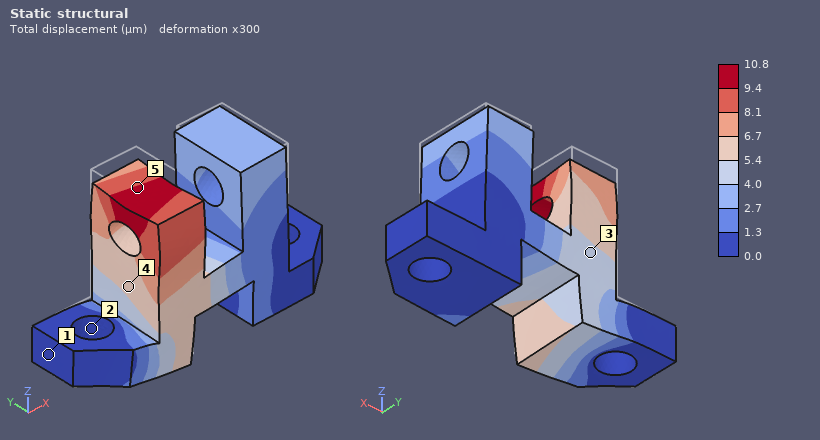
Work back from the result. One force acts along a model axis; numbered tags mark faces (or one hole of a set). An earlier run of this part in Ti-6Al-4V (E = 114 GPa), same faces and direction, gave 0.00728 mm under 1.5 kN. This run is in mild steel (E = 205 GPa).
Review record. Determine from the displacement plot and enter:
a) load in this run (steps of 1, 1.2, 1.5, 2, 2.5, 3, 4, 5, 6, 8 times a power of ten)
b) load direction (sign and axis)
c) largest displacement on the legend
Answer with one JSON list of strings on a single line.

["4 kN", "-Z", "10.8 µm"]
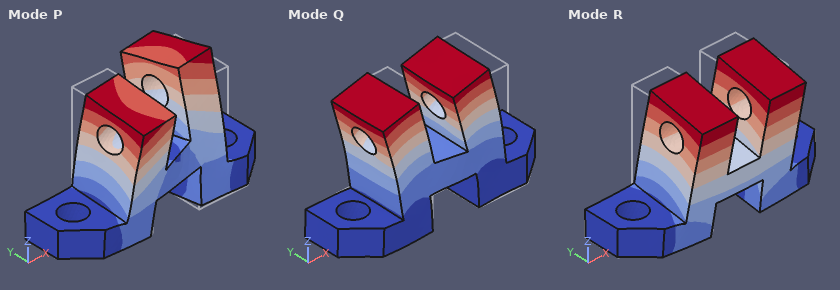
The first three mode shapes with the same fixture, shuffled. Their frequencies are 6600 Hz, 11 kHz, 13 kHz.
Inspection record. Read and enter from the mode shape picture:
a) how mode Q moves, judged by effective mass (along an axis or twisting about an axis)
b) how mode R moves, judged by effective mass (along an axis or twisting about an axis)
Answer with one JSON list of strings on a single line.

["along X", "along Y"]
